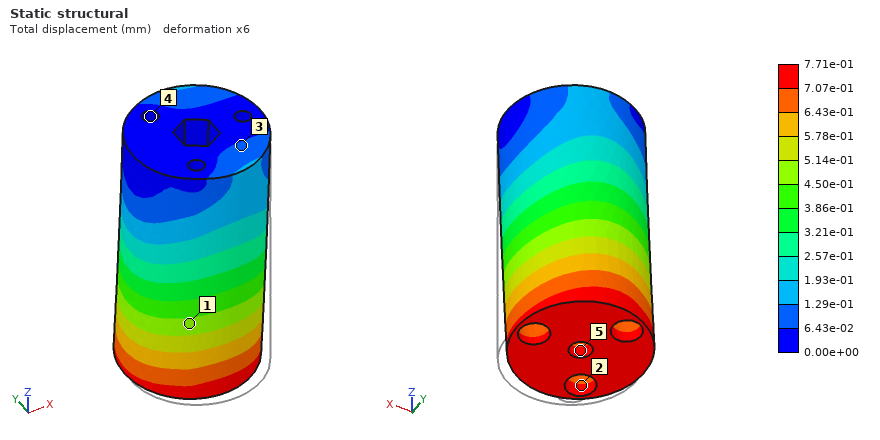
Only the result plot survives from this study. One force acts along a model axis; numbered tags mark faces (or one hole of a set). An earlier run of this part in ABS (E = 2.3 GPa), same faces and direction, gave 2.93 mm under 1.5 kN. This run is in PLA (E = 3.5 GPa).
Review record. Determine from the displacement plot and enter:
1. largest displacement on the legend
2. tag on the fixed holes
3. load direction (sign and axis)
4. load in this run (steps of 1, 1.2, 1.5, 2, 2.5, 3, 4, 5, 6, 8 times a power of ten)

7.71e-01 mm
4
+Y
600 N
